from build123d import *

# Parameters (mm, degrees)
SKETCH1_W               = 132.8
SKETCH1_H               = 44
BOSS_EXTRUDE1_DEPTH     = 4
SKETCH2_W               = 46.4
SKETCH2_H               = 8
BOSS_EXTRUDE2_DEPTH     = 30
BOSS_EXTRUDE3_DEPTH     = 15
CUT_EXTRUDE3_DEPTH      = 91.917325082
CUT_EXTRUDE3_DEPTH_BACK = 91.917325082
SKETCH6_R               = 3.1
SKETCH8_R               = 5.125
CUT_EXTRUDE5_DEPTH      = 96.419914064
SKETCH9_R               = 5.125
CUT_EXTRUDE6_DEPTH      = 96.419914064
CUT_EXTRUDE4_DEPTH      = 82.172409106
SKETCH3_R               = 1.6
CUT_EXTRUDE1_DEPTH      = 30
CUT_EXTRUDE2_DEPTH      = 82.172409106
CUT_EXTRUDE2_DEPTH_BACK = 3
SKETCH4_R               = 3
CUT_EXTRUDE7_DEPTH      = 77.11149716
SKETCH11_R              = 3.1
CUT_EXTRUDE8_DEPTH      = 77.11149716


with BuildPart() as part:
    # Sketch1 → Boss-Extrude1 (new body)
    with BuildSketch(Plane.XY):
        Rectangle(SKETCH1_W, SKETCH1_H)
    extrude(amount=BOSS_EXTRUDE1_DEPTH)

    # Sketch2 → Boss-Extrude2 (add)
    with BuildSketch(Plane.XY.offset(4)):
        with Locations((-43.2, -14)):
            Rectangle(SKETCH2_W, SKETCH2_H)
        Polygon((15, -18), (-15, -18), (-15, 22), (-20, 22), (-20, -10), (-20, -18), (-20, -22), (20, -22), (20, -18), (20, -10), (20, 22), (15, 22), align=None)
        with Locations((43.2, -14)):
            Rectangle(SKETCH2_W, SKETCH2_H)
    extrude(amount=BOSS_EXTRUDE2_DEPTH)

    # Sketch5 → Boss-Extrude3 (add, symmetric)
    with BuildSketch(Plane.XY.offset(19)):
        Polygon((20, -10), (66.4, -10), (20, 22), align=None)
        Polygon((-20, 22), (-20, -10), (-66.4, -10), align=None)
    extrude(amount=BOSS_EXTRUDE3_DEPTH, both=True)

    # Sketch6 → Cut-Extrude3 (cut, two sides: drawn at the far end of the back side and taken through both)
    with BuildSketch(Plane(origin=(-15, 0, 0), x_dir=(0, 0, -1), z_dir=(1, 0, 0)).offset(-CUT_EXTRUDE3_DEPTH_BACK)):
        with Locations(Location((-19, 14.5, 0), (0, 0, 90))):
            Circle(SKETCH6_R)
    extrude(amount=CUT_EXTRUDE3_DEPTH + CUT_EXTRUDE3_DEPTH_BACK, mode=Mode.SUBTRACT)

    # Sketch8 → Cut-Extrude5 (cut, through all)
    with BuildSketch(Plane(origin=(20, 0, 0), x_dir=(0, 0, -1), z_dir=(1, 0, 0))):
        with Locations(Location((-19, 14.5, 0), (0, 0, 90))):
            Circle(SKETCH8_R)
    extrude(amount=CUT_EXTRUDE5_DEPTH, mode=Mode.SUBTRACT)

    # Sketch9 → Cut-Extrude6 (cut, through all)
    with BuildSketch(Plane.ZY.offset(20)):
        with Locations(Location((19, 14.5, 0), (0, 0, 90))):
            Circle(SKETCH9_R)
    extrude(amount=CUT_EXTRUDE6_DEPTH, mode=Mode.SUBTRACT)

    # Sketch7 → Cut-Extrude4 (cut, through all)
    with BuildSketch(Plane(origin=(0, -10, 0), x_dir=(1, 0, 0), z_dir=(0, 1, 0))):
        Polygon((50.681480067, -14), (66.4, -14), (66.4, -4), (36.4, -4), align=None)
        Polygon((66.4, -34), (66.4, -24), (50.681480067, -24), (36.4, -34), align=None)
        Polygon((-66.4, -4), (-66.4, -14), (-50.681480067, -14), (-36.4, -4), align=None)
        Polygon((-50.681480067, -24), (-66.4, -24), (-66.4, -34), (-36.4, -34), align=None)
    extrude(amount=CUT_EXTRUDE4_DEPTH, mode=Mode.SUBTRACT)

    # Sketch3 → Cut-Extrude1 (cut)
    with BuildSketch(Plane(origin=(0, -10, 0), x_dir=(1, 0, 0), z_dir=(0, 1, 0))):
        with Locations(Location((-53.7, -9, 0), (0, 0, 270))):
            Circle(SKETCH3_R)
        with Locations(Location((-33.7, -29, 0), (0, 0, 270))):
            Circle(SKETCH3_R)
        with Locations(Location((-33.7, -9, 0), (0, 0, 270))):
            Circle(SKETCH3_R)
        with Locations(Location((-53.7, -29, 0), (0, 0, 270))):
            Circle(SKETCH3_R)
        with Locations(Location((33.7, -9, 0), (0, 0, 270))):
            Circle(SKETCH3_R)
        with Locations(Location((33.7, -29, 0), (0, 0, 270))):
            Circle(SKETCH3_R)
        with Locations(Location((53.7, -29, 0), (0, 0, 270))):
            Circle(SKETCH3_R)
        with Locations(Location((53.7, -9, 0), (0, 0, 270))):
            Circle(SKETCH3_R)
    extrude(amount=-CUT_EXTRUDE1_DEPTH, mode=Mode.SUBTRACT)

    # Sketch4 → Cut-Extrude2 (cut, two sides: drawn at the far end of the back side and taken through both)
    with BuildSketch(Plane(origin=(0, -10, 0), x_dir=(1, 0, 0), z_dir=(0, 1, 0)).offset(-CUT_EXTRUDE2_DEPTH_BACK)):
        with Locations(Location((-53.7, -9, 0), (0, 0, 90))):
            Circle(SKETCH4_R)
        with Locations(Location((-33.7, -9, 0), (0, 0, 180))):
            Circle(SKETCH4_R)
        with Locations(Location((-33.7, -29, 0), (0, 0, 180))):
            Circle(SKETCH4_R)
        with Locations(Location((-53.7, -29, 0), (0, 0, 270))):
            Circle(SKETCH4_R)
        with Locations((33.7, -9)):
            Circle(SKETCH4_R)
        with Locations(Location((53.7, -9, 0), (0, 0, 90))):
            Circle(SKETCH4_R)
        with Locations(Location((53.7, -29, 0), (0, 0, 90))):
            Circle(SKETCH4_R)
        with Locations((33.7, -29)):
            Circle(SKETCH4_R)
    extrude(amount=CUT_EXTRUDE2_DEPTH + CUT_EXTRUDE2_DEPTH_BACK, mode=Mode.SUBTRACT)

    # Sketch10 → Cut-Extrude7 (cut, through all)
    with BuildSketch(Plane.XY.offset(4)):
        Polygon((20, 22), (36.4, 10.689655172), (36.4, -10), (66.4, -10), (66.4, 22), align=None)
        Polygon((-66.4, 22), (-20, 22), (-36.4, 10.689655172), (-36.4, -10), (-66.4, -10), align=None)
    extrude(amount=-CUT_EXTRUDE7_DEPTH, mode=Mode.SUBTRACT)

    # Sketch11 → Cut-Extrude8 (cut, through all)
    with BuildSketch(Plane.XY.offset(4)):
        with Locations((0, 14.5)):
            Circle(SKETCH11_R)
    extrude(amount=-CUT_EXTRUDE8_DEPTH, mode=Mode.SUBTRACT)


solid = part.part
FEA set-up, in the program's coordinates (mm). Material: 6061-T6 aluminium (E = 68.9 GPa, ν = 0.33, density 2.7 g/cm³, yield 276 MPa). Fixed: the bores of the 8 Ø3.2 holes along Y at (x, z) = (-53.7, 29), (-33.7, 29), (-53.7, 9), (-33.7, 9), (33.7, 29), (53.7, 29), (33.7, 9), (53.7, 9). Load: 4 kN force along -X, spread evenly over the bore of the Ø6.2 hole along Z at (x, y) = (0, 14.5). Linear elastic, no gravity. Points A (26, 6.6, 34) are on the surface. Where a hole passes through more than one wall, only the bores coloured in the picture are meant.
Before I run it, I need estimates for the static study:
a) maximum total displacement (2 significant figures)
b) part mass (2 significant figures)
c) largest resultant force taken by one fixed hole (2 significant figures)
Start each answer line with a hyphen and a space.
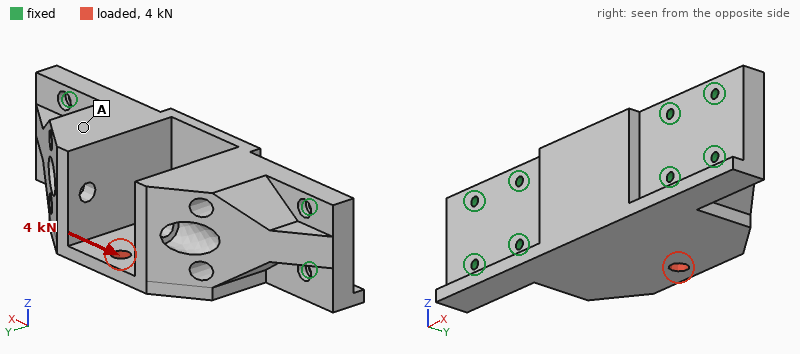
- 23 µm
- 230 g
- 1.4 kN
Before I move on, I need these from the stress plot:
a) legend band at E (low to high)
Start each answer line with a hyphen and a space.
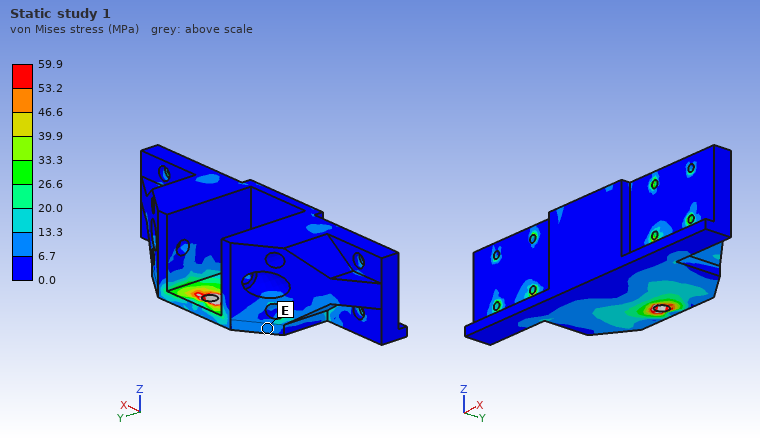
- 6.7 to 13.3 MPa
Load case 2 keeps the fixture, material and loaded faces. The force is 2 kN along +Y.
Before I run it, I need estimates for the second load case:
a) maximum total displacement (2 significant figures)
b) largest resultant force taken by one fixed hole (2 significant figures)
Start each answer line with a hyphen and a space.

- 19 µm
- 1.3 kN
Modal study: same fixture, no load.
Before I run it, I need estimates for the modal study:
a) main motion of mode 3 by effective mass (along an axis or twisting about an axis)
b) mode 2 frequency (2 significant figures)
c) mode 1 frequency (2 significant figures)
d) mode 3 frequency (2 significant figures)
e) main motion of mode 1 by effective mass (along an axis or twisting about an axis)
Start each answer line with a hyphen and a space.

- along Y
- 8600 Hz
- 7600 Hz
- 9800 Hz
- along Z
